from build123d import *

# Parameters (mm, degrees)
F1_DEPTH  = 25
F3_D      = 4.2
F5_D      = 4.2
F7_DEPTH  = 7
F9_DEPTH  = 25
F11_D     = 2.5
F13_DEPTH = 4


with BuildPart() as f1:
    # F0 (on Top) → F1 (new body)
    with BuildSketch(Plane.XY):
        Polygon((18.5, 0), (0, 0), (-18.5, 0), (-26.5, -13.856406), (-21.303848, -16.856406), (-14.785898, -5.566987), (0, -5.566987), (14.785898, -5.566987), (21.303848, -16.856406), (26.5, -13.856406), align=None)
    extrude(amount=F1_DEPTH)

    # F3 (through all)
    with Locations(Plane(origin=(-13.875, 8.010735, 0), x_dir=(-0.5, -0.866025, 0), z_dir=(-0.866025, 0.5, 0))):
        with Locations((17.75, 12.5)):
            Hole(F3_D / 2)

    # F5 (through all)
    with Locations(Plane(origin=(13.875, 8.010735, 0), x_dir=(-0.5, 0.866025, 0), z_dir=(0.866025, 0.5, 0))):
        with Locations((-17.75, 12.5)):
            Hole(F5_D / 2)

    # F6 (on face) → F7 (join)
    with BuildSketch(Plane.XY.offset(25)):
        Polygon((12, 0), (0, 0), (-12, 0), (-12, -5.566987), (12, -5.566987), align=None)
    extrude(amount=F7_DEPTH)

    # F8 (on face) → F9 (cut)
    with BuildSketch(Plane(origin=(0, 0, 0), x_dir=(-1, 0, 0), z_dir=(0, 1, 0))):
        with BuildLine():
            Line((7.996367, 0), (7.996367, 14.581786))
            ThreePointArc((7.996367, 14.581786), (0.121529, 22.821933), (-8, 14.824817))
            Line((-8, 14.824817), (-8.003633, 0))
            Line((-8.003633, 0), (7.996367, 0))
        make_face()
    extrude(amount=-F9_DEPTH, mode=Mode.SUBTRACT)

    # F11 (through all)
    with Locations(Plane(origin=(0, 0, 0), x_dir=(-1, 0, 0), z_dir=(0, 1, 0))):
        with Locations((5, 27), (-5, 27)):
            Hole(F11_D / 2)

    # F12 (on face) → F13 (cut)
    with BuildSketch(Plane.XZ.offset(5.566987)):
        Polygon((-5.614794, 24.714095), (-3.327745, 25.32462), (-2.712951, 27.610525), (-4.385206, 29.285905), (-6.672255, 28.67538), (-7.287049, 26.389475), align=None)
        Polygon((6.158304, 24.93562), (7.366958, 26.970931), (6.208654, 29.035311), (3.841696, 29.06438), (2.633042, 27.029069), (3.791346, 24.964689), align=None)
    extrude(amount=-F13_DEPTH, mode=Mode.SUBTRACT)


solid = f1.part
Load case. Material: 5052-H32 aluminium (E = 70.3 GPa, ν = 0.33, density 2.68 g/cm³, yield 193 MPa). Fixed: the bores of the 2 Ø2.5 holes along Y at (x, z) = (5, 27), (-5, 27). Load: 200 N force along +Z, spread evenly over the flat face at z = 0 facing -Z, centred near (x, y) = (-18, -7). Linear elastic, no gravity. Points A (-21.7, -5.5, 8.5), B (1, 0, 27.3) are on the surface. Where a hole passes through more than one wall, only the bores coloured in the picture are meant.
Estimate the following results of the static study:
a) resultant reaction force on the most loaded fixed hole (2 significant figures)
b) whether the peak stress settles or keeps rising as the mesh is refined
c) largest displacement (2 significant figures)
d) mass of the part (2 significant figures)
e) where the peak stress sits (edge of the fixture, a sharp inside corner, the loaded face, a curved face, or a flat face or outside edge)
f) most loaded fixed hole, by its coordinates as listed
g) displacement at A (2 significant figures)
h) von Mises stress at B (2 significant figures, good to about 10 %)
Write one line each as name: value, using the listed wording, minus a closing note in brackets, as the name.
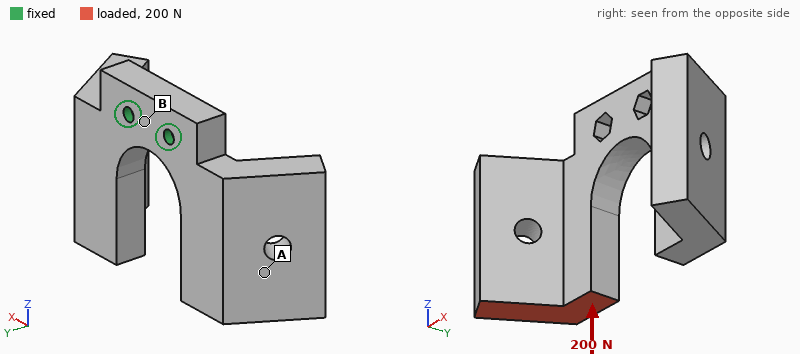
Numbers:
resultant reaction force on the most loaded fixed hole: 370 N
whether the peak stress settles or keeps rising as the mesh is refined: keeps rising
largest displacement: 0.11 mm
mass of the part: 21 g
where the peak stress sits: edge of the fixture
most loaded fixed hole, by its coordinates as listed: (-5, 27)
displacement at A: 0.067 mm
von Mises stress at B: 25 MPa
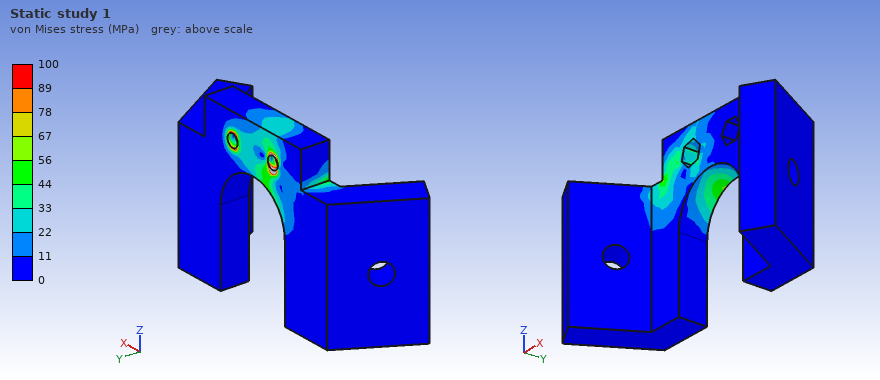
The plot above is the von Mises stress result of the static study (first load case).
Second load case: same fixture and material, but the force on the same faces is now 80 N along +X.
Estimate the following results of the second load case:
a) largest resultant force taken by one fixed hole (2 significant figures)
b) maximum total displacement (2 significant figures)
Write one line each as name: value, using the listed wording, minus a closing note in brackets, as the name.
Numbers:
largest resultant force taken by one fixed hole: 190 N
maximum total displacement: 52 µm
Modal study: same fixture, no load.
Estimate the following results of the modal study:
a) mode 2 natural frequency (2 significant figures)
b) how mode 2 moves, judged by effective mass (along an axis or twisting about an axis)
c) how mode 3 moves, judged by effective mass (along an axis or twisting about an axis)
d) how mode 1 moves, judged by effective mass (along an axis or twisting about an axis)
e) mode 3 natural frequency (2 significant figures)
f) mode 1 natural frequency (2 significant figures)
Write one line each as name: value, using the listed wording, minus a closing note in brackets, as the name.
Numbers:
mode 2 natural frequency: 2100 Hz
how mode 2 moves, judged by effective mass: twisting about Z
how mode 3 moves, judged by effective mass: along X
how mode 1 moves, judged by effective mass: along Y
mode 3 natural frequency: 3100 Hz
mode 1 natural frequency: 1600 Hz
